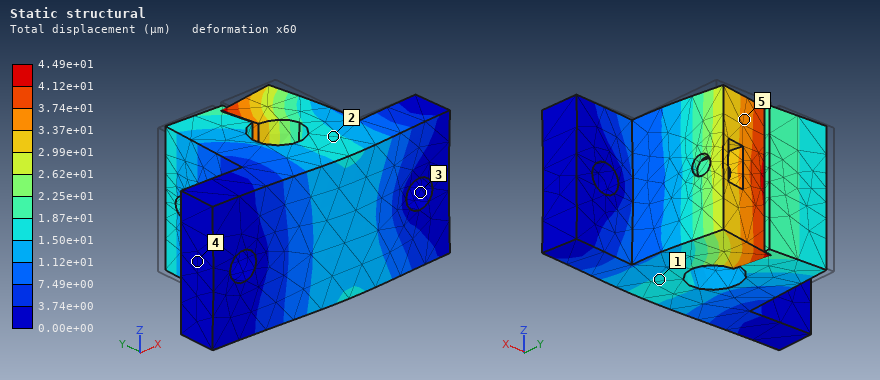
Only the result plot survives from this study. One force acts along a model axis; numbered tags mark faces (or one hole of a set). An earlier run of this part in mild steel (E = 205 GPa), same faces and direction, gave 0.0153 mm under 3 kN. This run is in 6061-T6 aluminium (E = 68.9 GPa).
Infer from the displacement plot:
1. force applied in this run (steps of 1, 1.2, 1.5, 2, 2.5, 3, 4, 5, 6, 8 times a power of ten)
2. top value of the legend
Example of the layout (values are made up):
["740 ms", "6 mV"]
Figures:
["3 kN", "4.49e+01 µm"]
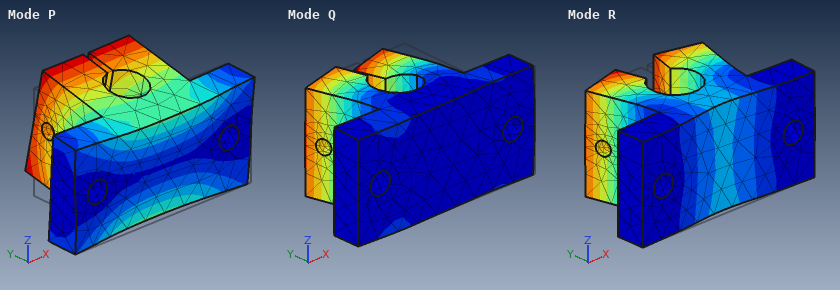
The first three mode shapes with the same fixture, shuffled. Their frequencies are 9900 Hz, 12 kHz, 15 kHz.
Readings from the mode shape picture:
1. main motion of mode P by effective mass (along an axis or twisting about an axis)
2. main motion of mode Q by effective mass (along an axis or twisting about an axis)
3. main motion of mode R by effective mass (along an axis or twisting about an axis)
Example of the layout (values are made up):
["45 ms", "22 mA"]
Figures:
["along Z", "along X", "along Y"]
